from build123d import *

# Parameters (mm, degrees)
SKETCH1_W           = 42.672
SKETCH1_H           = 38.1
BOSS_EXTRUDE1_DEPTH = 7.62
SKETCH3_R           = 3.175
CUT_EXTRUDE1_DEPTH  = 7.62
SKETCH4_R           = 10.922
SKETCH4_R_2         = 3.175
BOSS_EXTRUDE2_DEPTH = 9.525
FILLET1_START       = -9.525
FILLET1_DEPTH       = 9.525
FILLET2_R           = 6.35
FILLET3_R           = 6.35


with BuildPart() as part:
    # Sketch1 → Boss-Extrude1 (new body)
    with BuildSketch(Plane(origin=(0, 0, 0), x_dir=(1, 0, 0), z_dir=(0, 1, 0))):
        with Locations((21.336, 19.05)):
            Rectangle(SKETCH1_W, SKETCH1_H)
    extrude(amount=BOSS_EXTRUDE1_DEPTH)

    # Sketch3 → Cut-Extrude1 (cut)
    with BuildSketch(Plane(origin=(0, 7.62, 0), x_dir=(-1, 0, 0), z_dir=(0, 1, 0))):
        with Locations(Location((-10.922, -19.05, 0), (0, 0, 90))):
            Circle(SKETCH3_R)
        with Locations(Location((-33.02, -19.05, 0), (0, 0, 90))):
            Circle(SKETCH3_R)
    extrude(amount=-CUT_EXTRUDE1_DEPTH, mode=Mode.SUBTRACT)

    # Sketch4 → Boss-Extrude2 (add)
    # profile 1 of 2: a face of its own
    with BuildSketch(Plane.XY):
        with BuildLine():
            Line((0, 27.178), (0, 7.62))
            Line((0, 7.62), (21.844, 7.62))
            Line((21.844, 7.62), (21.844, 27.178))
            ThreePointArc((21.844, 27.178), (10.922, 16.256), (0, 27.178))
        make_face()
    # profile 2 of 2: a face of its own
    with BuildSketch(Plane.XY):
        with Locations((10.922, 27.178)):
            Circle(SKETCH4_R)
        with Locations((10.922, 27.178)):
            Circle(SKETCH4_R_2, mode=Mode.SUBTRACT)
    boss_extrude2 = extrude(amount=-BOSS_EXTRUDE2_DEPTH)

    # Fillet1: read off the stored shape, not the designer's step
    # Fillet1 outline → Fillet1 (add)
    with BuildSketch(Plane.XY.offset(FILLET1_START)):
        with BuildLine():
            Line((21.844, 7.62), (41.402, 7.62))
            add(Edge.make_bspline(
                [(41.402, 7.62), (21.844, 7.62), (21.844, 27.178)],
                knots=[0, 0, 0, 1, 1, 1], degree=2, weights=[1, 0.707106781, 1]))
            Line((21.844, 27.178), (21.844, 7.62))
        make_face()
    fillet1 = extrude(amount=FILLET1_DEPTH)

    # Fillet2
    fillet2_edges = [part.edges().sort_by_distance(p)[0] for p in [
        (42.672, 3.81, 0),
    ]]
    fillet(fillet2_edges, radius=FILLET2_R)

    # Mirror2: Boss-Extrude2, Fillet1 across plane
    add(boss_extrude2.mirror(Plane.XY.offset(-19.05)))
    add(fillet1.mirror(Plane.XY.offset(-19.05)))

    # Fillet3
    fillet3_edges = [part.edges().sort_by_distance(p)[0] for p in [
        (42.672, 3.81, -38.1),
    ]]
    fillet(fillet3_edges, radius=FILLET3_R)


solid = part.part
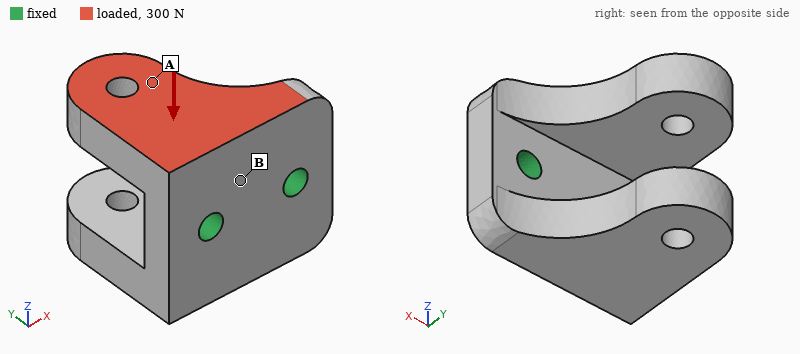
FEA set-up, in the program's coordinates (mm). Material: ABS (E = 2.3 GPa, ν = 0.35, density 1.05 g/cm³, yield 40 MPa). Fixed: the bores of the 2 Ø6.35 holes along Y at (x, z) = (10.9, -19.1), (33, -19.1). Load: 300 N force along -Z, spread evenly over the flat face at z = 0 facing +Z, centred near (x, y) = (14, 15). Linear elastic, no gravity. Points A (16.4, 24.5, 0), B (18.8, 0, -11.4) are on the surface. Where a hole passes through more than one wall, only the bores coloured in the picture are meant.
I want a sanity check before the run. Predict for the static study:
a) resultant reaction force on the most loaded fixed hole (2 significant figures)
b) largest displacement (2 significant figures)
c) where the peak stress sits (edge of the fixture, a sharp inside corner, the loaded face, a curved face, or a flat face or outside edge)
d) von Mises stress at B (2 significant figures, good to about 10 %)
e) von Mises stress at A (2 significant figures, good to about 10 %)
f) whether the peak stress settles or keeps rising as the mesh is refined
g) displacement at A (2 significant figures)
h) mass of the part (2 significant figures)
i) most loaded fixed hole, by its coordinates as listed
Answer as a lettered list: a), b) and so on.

a) 240 N
b) 0.65 mm
c) edge of the fixture
d) 6.9 MPa
e) 2.2 MPa
f) keeps rising
g) 0.39 mm
h) 26 g
i) (10.9, -19.1)
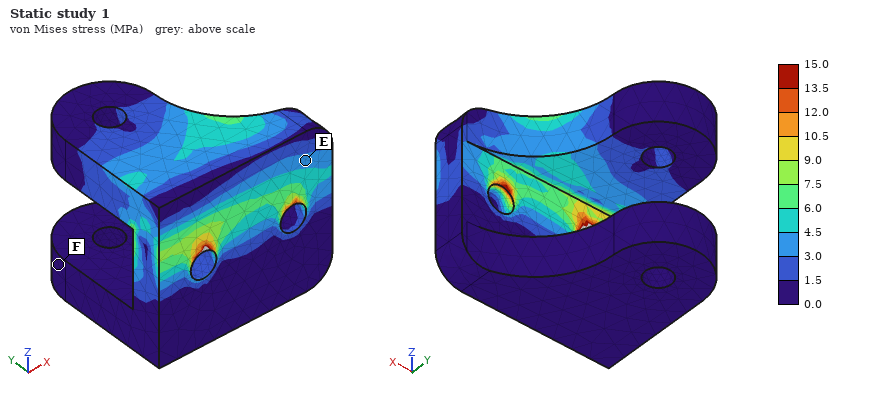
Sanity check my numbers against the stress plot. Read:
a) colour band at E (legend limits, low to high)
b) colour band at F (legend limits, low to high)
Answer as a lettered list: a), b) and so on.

a) 3.0 to 4.5 MPa
b) 0.0 to 1.5 MPa
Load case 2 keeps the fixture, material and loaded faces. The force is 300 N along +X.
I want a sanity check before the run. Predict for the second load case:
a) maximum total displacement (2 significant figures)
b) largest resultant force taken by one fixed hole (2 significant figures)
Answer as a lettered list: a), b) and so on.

a) 0.17 mm
b) 290 N
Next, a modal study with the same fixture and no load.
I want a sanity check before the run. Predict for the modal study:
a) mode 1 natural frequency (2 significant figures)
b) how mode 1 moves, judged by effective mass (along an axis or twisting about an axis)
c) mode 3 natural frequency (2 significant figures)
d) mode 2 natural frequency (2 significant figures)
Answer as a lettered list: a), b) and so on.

a) 1300 Hz
b) along Z
c) 2500 Hz
d) 1400 Hz
